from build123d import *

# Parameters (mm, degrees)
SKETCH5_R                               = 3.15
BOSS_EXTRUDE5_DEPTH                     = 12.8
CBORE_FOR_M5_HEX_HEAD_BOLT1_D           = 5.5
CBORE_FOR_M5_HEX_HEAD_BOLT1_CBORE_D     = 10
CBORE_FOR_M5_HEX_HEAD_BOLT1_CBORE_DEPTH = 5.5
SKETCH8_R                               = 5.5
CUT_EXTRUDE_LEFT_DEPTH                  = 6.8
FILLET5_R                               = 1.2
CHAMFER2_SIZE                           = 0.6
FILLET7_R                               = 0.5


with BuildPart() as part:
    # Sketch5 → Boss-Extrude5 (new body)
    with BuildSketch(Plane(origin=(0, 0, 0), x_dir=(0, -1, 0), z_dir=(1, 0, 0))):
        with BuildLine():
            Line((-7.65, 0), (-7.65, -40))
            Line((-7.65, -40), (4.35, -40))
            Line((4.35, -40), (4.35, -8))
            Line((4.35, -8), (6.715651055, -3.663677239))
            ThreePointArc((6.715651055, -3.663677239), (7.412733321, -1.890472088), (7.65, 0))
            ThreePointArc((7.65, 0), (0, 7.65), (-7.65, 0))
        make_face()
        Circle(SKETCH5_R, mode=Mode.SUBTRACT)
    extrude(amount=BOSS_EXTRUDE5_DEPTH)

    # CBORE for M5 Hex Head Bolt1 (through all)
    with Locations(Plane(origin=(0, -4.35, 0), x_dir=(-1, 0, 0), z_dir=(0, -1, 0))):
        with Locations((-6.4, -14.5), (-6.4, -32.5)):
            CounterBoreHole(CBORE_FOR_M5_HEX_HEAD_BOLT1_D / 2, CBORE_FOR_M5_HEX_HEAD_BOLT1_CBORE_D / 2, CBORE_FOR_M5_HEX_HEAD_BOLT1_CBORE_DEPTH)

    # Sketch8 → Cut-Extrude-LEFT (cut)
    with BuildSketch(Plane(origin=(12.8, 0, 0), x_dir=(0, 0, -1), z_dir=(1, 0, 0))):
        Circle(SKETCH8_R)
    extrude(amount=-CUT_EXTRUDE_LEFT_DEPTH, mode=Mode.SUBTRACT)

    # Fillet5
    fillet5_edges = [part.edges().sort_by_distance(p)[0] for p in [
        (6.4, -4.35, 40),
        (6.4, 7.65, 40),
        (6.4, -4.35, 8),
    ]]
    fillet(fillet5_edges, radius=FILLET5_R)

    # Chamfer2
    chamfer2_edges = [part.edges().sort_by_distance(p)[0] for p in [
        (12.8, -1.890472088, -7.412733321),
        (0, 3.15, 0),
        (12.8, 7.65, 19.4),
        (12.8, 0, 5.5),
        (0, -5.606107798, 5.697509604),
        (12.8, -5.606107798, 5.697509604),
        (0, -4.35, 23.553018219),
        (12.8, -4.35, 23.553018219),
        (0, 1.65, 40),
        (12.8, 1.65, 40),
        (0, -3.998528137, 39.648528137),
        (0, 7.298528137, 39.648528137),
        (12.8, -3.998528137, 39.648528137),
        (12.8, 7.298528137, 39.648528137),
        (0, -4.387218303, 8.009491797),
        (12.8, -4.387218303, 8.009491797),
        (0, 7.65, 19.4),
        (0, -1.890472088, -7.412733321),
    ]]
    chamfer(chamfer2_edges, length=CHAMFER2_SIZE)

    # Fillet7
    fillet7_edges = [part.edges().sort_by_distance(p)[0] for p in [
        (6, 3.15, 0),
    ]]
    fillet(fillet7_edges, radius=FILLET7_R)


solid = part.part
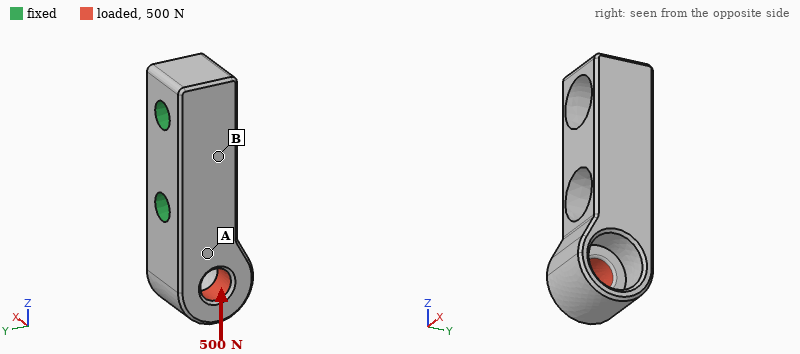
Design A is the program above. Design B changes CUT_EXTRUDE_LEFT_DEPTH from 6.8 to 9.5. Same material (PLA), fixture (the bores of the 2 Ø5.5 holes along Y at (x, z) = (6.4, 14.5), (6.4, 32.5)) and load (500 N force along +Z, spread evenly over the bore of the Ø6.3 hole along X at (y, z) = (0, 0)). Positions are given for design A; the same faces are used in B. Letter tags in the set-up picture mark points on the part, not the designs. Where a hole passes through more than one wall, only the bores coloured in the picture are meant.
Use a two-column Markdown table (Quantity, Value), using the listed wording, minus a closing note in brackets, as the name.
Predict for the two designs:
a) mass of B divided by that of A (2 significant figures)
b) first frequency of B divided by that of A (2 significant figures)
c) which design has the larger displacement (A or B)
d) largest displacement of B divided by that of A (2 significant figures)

| Quantity | Value |
|---|---|
| mass of B divided by that of A | 0.97 |
| first frequency of B divided by that of A | 1.00 |
| which design has the larger displacement | B |
| largest displacement of B divided by that of A | 1.3 |
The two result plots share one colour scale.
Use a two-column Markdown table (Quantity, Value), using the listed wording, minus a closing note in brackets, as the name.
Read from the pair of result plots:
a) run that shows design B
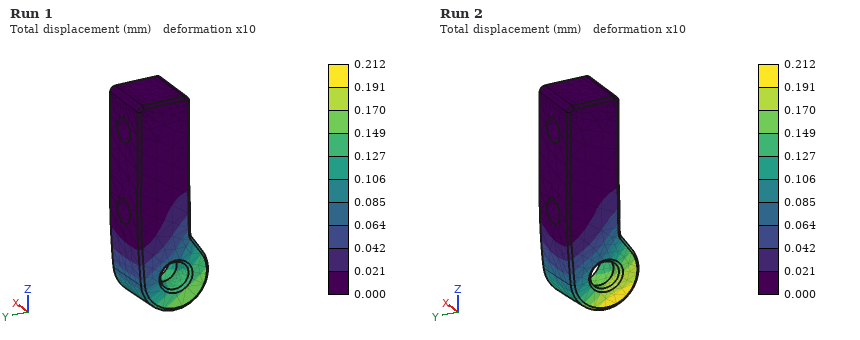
| Quantity | Value |
|---|---|
| run that shows design B | Run 2 |
